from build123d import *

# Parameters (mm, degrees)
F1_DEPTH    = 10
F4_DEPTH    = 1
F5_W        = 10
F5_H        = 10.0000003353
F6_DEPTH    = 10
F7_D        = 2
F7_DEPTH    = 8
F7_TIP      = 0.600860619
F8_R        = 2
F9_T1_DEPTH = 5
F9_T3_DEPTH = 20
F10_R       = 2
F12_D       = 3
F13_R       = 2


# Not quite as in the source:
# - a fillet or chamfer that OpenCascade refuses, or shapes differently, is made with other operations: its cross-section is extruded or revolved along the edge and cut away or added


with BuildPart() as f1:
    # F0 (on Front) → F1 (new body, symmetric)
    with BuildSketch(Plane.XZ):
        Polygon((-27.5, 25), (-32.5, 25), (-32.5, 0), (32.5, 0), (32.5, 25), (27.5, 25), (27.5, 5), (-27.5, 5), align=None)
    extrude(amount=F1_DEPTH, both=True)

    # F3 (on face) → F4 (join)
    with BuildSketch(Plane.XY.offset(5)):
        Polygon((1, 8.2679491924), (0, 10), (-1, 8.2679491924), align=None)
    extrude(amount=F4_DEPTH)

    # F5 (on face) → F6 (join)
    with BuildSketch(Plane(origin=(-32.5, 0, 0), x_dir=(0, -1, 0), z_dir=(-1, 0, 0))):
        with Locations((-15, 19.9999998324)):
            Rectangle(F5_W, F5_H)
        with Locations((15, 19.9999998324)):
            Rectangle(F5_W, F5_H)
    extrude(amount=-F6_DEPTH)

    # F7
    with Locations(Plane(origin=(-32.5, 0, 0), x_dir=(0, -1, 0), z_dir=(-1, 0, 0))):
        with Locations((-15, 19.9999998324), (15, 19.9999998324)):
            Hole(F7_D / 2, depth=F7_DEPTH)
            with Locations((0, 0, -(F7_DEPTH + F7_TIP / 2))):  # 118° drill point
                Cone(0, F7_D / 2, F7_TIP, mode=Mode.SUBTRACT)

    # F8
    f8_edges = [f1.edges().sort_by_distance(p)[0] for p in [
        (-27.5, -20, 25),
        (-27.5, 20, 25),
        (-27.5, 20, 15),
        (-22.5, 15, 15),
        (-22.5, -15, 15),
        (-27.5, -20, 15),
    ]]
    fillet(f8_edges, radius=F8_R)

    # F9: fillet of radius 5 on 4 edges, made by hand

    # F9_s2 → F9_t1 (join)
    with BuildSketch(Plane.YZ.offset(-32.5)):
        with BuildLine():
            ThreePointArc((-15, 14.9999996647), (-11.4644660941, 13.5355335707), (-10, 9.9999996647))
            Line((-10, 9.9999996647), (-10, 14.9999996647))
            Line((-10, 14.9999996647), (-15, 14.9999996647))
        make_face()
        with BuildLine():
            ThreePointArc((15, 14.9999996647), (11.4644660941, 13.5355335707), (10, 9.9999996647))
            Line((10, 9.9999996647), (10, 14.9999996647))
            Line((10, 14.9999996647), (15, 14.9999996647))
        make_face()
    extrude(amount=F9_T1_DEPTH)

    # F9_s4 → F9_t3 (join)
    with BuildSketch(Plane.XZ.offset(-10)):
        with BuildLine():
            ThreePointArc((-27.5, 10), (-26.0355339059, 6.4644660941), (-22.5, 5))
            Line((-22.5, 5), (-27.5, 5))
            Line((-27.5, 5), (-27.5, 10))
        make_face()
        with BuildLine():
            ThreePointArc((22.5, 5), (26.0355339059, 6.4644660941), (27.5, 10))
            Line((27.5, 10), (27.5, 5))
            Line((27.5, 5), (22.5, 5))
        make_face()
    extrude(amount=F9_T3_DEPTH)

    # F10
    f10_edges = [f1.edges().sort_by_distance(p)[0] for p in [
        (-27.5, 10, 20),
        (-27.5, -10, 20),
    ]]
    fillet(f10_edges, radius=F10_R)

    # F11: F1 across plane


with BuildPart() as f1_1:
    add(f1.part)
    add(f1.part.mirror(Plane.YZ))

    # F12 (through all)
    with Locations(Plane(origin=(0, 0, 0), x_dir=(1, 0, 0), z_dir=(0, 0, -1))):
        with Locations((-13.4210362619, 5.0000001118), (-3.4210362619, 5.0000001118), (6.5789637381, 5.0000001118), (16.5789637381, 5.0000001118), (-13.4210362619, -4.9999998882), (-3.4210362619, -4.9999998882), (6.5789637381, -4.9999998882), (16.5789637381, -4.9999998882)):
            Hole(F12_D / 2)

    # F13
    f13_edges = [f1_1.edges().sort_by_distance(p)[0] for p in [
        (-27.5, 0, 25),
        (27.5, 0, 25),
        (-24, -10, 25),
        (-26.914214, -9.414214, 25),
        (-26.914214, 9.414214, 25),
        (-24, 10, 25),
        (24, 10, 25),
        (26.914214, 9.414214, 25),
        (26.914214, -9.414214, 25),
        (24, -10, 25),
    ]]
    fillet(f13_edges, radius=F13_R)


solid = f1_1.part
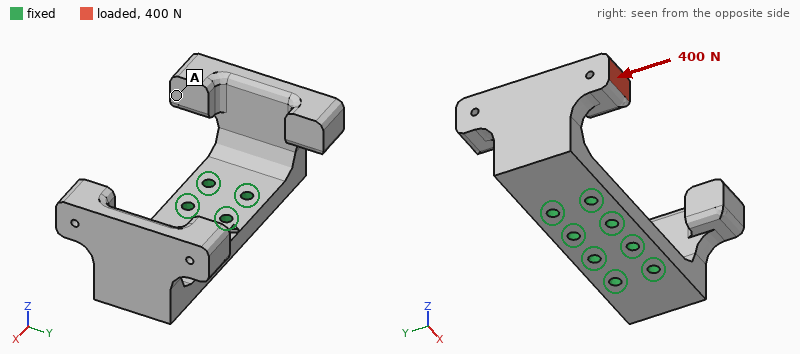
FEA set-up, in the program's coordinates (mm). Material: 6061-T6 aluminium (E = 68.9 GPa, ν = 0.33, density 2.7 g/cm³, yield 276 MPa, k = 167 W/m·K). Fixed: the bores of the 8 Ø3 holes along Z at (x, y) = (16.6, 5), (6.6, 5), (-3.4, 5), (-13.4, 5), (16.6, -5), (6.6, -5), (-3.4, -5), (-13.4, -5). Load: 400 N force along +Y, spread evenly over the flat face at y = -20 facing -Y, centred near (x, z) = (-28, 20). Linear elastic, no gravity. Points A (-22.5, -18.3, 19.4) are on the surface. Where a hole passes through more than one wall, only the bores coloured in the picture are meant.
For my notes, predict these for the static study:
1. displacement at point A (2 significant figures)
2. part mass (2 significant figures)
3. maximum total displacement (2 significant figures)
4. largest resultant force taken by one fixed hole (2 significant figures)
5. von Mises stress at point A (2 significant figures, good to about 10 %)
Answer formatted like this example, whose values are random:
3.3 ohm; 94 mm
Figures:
0.097 mm; 39 g; 0.11 mm; 650 N; 6.6 MPa
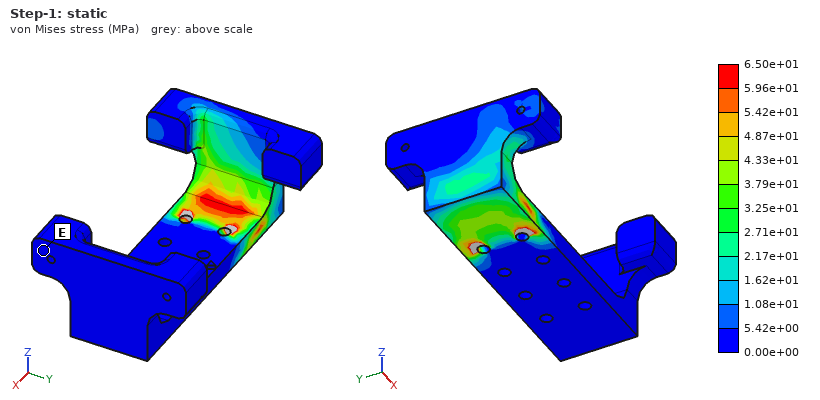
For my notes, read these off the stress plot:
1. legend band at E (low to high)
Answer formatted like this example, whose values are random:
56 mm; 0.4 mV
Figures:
0.00e+00 to 5.42e+00 MPa
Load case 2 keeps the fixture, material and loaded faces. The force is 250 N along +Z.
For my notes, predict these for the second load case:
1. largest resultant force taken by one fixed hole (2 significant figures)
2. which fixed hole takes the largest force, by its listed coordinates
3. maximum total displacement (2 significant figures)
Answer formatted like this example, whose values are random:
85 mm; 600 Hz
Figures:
510 N; (-13.4, -5); 99 µm
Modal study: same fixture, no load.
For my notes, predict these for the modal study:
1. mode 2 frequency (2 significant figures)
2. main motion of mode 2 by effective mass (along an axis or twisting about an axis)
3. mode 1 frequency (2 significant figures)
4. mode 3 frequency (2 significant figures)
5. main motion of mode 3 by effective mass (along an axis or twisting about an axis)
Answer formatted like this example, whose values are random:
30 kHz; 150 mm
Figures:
3100 Hz; along X; 2600 Hz; 3500 Hz; along Y
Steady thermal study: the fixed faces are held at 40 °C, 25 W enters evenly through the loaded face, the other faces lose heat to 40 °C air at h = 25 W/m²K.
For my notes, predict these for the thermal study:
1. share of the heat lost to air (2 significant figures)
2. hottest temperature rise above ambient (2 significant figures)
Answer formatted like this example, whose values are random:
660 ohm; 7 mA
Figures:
8.7 %; 68 K
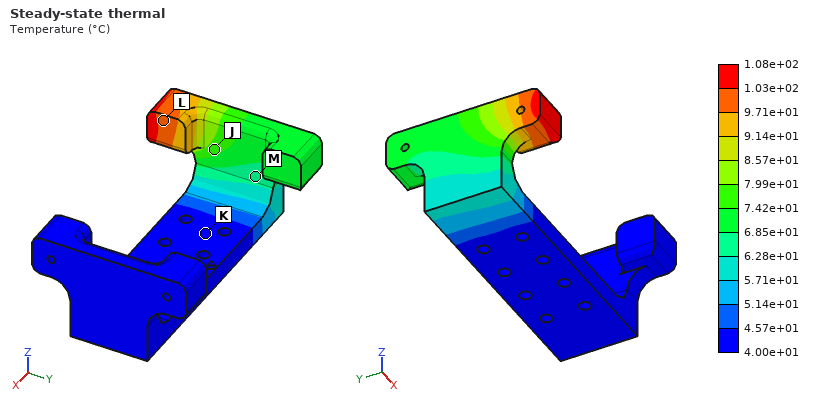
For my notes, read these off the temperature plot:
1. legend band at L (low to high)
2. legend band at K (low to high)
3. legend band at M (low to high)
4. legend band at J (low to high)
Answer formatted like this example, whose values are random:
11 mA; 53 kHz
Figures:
9.71e+01 to 1.03e+02 °C; 4.00e+01 to 4.57e+01 °C; 6.28e+01 to 6.85e+01 °C; 7.42e+01 to 7.99e+01 °C
